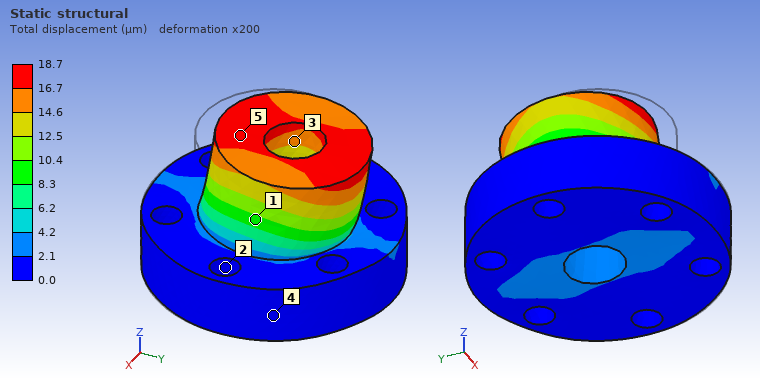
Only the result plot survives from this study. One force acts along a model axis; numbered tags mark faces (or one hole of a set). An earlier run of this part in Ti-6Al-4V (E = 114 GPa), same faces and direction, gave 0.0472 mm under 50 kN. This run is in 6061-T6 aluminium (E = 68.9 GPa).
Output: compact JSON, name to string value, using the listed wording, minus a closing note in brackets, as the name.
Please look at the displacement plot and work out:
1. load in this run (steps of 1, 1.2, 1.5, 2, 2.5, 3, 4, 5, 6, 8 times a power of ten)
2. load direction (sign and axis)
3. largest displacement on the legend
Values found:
{"load in this run": "12 kN", "load direction": "+Y", "largest displacement on the legend": "18.7 µm"}
